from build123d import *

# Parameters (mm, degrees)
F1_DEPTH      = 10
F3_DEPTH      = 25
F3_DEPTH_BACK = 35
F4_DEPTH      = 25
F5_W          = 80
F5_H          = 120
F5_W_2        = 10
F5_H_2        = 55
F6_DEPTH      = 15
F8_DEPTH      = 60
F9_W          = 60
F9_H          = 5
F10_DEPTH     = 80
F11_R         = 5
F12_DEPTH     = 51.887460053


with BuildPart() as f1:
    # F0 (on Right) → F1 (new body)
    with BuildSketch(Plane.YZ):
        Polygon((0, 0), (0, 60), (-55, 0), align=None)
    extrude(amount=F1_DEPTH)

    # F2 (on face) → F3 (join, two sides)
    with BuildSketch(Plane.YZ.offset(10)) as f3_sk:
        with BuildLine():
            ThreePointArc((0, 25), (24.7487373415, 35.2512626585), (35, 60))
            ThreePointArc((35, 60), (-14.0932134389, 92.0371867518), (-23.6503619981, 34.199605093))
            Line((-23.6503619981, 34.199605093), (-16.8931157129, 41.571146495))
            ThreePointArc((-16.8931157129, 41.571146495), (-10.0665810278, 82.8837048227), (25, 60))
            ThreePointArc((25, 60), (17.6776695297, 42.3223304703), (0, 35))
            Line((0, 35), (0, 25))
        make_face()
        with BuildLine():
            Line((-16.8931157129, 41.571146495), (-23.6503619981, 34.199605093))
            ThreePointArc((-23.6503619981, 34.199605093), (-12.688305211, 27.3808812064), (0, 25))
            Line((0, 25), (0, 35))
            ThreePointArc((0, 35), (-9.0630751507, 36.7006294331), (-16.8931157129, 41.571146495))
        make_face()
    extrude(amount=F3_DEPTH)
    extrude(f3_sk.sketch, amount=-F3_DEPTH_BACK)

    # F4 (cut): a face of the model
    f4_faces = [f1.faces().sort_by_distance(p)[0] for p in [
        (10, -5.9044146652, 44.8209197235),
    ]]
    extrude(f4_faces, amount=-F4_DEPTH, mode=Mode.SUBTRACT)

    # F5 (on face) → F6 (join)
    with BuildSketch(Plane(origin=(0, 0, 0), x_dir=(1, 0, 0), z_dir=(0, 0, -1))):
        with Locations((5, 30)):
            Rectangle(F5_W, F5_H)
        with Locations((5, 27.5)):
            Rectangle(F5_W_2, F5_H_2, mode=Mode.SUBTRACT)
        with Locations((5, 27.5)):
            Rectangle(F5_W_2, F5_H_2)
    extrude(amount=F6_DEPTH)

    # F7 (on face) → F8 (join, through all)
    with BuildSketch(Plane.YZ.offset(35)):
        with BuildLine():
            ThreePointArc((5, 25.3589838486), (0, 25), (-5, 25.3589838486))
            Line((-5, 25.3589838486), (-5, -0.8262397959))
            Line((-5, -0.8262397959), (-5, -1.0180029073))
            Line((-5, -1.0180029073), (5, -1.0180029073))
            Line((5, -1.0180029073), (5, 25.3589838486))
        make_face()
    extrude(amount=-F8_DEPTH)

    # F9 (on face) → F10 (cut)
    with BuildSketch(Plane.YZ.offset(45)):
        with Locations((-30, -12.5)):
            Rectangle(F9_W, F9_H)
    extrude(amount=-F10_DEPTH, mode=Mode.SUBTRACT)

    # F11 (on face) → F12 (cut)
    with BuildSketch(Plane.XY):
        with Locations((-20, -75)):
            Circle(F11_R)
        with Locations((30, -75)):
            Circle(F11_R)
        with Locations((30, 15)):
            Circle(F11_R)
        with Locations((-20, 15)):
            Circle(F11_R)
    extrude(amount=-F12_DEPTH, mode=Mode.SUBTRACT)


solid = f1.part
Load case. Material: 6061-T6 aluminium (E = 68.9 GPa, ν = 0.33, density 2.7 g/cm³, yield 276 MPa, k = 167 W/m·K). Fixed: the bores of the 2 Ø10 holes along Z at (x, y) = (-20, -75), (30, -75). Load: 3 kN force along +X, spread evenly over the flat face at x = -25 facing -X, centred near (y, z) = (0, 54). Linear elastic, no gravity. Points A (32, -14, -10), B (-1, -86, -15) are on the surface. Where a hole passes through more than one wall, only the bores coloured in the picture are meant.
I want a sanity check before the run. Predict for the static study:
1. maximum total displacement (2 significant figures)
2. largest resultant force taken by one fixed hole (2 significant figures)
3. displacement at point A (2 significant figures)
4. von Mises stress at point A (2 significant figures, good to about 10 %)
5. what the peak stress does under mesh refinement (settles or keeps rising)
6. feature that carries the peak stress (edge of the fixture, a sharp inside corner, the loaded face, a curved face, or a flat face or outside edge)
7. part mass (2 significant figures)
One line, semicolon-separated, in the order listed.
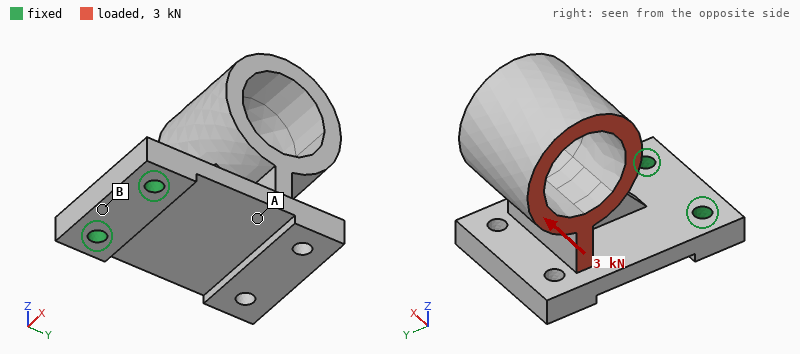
0.87 mm; 5.4 kN; 0.18 mm; 53 MPa; keeps rising; edge of the fixture; 690 g
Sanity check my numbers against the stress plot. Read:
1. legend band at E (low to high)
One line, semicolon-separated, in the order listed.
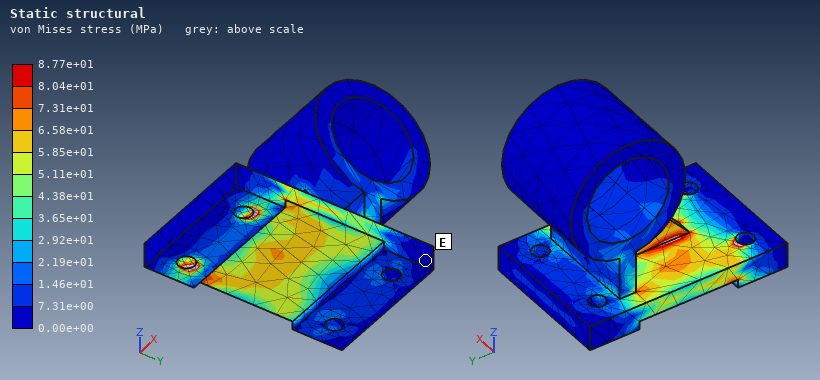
0.00e+00 to 7.31e+00 MPa
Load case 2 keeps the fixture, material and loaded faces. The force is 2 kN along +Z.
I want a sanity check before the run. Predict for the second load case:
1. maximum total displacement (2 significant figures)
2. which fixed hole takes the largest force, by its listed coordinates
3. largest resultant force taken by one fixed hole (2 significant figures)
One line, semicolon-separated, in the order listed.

0.87 mm; (-20, -75); 2.1 kN
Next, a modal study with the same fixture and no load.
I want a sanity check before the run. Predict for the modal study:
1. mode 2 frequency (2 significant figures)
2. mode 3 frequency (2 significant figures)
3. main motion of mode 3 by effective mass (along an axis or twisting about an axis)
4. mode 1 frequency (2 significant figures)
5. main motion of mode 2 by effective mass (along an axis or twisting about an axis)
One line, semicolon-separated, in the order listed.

580 Hz; 1800 Hz; along Z; 360 Hz; along X
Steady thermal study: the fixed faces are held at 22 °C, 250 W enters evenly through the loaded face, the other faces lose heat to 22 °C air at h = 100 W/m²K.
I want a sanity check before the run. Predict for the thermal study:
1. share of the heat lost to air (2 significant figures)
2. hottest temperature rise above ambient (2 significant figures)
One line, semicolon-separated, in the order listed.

76 %; 76 K
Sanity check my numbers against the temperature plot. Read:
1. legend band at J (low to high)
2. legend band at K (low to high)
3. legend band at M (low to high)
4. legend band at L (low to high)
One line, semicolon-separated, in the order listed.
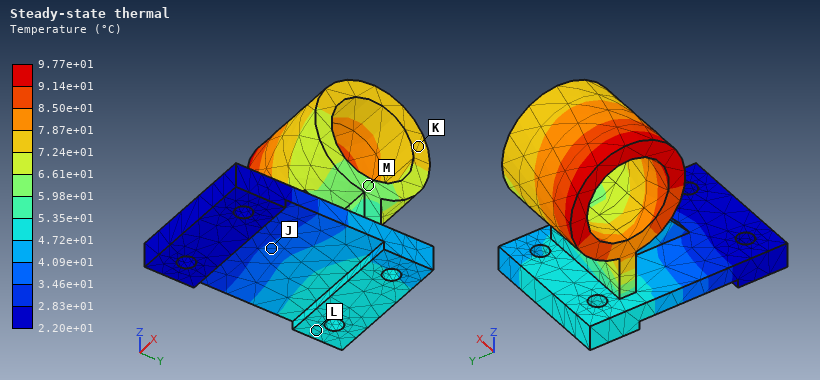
3.46e+01 to 4.09e+01 °C; 7.24e+01 to 7.87e+01 °C; 5.98e+01 to 6.61e+01 °C; 4.72e+01 to 5.35e+01 °C
